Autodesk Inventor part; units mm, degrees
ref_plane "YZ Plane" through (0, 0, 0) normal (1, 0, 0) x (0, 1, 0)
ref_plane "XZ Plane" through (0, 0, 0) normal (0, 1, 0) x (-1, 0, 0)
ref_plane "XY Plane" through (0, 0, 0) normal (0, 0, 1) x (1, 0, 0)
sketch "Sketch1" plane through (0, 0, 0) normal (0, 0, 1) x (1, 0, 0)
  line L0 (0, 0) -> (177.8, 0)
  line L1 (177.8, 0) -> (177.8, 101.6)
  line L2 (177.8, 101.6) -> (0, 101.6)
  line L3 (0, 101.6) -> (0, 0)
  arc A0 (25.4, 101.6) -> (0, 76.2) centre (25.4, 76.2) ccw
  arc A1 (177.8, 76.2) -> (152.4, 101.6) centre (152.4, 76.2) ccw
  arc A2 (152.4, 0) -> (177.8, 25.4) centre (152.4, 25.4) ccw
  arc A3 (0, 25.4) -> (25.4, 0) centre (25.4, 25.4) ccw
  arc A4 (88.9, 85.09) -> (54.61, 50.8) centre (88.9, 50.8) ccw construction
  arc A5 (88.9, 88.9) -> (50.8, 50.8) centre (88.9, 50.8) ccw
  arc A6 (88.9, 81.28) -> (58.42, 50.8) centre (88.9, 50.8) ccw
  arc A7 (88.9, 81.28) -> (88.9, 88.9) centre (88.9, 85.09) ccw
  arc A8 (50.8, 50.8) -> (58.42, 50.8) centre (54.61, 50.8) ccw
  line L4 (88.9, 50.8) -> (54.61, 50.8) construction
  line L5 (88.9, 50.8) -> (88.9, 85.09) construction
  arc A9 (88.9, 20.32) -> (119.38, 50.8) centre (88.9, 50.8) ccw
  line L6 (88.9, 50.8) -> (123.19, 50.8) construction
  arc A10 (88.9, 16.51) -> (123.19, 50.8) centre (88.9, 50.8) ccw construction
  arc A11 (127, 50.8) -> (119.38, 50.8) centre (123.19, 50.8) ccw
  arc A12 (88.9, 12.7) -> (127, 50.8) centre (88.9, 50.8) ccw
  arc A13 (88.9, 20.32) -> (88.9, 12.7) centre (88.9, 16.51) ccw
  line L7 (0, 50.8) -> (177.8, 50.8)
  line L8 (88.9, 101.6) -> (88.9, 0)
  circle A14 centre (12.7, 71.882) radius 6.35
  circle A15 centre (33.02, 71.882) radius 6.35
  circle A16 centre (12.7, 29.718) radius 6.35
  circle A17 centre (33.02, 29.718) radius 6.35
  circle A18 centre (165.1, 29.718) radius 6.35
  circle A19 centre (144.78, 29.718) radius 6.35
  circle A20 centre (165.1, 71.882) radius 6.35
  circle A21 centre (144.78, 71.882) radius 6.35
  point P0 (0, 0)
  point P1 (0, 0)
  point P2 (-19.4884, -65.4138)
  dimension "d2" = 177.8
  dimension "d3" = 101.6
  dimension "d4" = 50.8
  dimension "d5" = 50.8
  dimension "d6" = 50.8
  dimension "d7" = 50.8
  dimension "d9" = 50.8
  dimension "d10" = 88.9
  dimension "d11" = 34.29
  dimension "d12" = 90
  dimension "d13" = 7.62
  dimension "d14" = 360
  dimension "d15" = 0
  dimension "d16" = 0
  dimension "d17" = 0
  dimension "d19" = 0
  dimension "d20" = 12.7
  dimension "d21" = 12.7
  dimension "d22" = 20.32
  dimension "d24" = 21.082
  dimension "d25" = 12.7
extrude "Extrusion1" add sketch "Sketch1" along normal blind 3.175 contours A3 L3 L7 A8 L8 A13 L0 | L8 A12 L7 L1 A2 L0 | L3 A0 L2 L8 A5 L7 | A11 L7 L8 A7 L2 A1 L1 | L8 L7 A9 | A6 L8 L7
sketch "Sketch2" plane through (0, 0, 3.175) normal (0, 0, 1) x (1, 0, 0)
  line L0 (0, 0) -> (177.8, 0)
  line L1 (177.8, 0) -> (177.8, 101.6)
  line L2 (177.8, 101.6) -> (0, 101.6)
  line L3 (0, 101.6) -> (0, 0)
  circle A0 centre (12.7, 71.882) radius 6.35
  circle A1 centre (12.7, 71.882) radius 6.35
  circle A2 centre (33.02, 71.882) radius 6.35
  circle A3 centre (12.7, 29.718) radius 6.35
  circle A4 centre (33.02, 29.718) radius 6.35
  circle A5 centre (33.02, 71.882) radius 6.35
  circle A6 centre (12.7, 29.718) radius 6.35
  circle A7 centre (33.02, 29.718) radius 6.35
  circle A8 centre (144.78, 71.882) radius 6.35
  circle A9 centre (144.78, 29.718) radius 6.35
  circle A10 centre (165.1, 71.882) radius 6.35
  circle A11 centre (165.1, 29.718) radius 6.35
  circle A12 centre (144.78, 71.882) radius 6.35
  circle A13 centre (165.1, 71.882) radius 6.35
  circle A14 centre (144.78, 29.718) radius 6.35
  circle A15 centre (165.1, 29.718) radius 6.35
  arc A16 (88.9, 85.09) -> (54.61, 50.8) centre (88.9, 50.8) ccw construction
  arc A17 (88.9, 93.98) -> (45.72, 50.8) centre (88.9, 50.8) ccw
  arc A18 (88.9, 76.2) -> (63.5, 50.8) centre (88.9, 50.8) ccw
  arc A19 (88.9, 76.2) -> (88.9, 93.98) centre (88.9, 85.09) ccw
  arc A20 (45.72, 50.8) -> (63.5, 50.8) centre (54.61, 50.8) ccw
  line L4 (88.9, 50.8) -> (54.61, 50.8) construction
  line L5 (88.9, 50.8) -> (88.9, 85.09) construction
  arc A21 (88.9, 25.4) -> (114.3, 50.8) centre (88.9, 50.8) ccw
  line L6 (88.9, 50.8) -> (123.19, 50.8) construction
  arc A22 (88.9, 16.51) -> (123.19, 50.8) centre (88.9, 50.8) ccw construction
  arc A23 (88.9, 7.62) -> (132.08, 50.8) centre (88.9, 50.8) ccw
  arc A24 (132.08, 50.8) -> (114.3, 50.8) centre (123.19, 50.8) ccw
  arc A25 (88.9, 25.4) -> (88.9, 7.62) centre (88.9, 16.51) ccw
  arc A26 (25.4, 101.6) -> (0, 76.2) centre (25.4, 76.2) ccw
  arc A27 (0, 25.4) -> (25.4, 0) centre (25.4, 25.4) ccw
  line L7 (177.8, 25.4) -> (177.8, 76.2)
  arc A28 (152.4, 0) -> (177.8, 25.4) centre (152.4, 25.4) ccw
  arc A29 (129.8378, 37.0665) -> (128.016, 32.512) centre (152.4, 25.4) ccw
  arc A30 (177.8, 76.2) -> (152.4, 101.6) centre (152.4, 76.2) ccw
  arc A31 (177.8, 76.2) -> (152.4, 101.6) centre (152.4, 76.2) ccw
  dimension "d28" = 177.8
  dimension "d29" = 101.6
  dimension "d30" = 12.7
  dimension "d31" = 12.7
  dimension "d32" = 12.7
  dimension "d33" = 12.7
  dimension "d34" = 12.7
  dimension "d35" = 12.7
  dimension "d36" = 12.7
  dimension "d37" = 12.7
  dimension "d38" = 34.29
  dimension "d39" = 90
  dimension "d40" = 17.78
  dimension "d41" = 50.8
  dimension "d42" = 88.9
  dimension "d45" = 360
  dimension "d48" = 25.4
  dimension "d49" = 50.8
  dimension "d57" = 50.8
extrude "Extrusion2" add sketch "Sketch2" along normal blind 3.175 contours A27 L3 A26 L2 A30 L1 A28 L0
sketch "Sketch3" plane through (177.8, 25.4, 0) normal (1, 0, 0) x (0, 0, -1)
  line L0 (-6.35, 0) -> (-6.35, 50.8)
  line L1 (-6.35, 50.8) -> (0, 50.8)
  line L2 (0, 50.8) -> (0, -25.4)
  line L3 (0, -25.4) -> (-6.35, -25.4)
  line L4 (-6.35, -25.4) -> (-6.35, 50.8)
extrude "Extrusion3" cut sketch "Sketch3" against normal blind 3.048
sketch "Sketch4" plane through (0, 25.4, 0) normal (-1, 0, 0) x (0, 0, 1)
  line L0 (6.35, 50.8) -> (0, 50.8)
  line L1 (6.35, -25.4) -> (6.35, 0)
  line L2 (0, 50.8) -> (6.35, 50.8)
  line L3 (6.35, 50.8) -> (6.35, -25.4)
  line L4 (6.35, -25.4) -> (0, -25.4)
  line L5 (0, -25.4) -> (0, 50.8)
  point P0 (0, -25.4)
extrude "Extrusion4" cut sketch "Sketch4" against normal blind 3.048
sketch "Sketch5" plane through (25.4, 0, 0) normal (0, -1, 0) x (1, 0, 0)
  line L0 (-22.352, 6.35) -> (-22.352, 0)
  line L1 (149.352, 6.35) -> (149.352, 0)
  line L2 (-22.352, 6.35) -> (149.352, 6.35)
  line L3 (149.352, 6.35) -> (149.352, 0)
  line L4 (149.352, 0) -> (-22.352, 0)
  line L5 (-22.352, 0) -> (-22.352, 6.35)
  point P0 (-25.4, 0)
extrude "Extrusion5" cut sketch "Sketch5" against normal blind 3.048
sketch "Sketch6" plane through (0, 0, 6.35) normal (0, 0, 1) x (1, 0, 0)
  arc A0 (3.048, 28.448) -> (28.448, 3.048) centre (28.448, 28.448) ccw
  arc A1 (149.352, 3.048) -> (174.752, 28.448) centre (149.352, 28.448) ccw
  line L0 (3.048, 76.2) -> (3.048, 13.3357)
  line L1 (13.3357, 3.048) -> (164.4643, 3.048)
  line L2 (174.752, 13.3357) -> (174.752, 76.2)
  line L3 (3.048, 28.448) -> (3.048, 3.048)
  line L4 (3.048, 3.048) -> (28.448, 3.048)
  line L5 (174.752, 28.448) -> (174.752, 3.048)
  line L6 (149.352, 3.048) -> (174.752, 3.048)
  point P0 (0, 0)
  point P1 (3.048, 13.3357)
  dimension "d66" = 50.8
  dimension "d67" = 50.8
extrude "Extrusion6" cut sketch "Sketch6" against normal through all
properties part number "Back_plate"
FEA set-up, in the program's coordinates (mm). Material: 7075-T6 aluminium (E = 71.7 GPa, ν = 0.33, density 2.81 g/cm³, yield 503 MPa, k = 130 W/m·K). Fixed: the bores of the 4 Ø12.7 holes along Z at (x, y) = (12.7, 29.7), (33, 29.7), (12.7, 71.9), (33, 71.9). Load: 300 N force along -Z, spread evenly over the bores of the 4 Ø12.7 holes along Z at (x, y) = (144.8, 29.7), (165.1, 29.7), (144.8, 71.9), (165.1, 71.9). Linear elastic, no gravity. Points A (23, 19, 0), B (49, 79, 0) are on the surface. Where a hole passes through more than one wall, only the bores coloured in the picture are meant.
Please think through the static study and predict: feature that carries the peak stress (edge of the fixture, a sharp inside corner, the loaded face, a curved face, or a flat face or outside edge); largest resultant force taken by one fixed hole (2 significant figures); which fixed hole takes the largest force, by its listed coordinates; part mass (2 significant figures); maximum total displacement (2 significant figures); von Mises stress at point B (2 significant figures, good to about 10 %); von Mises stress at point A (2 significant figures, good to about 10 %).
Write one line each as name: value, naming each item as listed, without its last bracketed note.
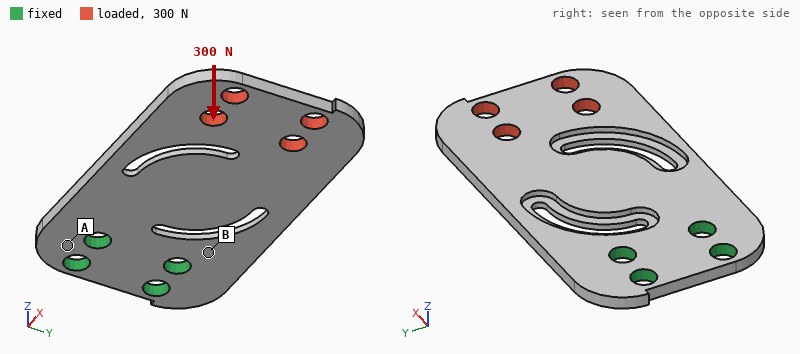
feature that carries the peak stress: a curved face
largest resultant force taken by one fixed hole: 490 N
which fixed hole takes the largest force, by its listed coordinates: (33, 29.7)
part mass: 250 g
maximum total displacement: 2.3 mm
von Mises stress at point B: 45 MPa
von Mises stress at point A: 10 MPa
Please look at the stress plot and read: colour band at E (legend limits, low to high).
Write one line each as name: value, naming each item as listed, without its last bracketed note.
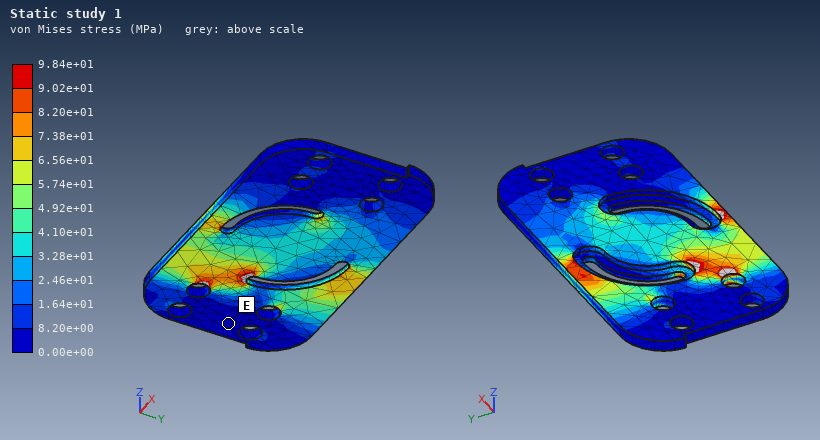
colour band at E: 0.00e+00 to 8.20e+00 MPa
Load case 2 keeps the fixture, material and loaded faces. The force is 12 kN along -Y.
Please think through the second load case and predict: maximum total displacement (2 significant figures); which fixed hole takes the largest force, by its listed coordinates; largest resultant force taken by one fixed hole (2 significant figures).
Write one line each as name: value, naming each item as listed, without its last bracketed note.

maximum total displacement: 0.83 mm
which fixed hole takes the largest force, by its listed coordinates: (33, 29.7)
largest resultant force taken by one fixed hole: 21 kN
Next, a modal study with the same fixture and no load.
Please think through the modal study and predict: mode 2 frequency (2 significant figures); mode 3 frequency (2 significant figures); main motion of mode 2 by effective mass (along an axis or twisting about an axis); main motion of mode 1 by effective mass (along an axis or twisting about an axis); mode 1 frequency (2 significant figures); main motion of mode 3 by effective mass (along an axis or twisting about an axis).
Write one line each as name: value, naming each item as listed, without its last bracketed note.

mode 2 frequency: 740 Hz
mode 3 frequency: 1500 Hz
main motion of mode 2 by effective mass: twisting about X
main motion of mode 1 by effective mass: along Z
mode 1 frequency: 240 Hz
main motion of mode 3 by effective mass: along Z
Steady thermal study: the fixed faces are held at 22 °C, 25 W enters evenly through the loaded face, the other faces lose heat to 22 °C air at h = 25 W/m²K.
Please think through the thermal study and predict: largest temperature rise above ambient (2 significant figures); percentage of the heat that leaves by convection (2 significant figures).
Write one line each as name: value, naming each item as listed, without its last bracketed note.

largest temperature rise above ambient: 39 K
percentage of the heat that leaves by convection: 53 %
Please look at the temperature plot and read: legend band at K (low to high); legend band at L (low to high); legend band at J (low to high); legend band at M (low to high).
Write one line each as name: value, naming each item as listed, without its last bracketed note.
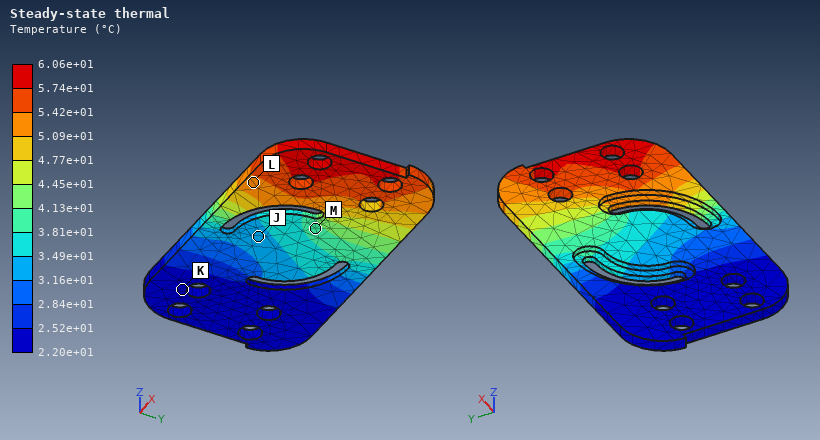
legend band at K: 2.20e+01 to 2.52e+01 °C
legend band at L: 5.09e+01 to 5.42e+01 °C
legend band at J: 3.16e+01 to 3.49e+01 °C
legend band at M: 3.81e+01 to 4.13e+01 °C
